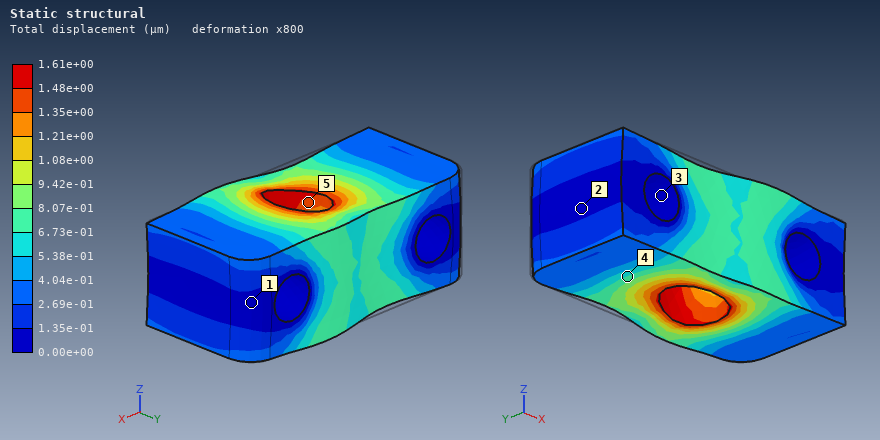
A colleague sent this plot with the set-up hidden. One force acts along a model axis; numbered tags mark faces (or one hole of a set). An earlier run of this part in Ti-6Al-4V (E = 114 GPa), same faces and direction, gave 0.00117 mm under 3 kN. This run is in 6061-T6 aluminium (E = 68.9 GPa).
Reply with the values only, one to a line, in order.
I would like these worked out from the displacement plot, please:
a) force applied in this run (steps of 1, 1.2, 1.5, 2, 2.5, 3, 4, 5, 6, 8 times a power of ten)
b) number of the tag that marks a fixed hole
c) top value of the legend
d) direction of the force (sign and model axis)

2.5 kN
3
1.61e+00 µm
+X
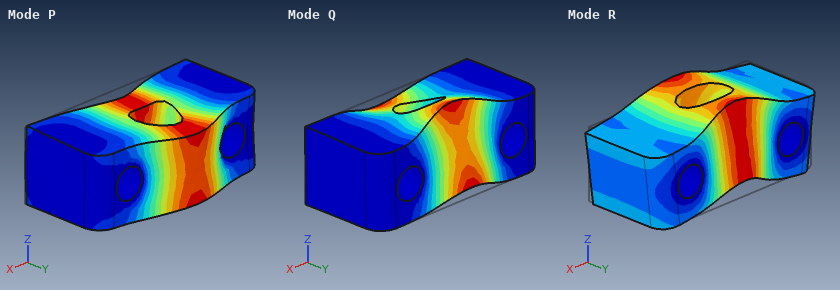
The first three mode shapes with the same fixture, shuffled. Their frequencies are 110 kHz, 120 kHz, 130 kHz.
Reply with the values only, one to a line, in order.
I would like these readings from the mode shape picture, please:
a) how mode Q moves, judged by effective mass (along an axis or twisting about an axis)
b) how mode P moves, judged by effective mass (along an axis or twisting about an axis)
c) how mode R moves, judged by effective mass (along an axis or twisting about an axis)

twisting about X
along Y
along Z
